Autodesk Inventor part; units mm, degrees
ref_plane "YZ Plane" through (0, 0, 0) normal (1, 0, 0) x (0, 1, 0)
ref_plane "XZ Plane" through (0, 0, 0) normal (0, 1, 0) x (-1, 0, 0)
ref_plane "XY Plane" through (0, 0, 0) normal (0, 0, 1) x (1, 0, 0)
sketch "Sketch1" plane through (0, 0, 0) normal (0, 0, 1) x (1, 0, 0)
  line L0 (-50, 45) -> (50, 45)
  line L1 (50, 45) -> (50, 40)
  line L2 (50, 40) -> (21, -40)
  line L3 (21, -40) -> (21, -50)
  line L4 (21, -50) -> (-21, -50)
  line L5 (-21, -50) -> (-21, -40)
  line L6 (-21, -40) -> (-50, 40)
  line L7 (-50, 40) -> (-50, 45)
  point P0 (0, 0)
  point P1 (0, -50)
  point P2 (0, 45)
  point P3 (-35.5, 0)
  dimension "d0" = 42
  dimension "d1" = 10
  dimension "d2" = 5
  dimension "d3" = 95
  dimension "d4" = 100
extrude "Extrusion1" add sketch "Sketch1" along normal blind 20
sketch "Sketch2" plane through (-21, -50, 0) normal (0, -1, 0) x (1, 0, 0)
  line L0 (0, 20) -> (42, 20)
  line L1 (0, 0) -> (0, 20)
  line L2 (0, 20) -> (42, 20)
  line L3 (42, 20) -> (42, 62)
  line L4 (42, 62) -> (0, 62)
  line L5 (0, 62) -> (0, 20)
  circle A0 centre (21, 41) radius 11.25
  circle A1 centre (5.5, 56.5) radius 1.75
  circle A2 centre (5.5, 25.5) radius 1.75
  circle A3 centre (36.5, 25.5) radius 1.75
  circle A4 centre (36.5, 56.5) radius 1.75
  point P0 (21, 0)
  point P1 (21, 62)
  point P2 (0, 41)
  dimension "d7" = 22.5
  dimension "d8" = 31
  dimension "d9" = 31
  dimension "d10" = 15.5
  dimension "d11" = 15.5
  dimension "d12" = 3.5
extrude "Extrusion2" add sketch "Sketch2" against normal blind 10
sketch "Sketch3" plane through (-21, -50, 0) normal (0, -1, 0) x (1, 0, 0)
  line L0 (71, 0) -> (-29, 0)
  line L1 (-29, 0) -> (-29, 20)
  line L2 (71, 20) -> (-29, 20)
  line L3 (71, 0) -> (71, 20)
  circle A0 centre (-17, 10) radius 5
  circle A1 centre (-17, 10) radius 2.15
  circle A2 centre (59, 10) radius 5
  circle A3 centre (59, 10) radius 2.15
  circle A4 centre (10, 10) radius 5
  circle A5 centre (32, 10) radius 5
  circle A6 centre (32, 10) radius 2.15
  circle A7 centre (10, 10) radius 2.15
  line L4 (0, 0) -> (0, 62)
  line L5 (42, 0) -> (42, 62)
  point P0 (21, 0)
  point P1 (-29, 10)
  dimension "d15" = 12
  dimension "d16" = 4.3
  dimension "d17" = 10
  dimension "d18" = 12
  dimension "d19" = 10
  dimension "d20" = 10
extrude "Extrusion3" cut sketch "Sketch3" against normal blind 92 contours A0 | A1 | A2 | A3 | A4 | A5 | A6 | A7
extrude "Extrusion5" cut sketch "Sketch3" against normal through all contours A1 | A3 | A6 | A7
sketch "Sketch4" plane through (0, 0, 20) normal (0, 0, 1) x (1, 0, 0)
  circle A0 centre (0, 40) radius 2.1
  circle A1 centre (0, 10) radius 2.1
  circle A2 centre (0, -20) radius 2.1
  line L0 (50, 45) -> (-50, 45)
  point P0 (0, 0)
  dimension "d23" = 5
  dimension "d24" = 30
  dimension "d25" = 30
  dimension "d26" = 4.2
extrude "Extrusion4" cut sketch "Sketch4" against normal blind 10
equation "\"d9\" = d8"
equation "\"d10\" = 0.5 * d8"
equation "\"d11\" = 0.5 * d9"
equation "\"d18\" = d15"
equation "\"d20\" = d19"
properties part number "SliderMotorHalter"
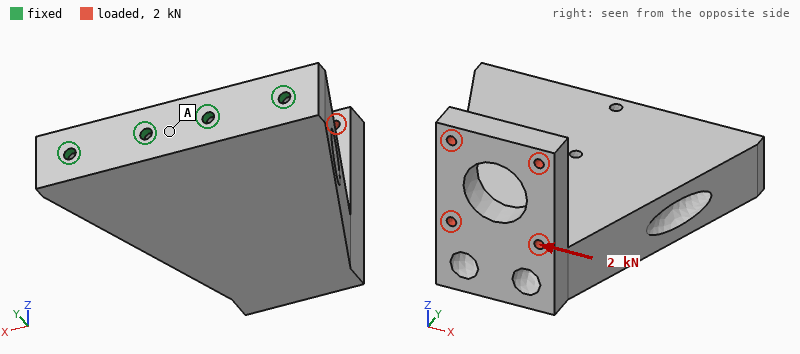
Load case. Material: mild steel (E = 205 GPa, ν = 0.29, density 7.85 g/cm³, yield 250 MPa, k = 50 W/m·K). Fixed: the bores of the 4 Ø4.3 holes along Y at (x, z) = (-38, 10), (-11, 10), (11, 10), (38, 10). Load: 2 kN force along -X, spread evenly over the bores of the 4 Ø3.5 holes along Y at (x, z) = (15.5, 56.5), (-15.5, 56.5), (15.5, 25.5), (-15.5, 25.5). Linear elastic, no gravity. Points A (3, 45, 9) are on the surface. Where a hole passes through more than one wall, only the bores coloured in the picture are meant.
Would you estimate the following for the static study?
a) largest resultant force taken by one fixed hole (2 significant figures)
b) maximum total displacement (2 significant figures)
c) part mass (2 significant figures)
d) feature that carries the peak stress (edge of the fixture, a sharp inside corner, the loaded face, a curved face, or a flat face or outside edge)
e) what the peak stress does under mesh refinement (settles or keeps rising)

2.3 kN
54 µm
980 g
edge of the fixture
keeps rising
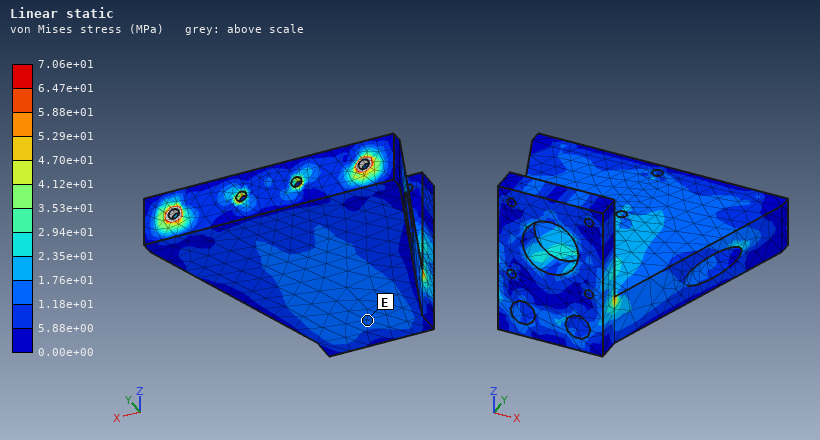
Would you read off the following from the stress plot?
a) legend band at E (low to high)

1.18e+01 to 1.76e+01 MPa
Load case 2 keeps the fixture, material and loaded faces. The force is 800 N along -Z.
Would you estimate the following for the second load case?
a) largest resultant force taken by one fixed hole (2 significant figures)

360 N
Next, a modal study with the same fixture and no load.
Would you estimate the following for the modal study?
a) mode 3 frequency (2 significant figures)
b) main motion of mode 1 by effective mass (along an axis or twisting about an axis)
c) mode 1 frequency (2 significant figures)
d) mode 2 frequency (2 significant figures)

3000 Hz
along Z
510 Hz
2900 Hz
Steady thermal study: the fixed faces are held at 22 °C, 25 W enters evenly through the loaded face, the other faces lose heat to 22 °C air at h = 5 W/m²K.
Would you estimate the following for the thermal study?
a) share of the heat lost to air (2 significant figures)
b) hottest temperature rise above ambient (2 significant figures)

17 %
89 K
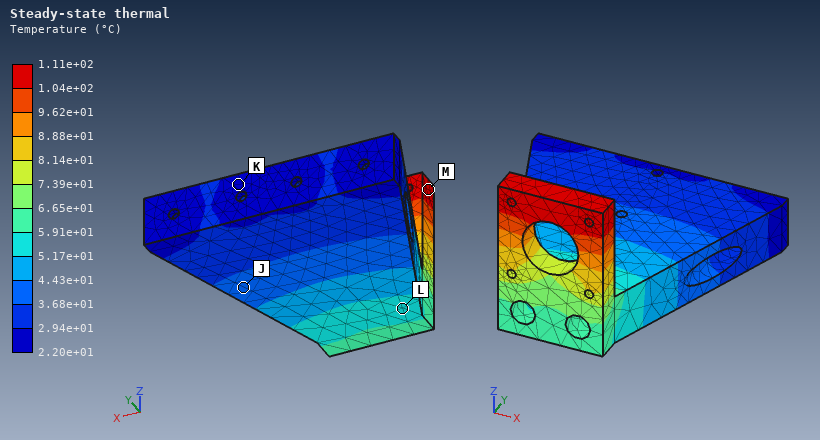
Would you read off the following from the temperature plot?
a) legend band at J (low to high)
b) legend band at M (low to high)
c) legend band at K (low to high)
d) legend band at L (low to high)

3.68e+01 to 4.43e+01 °C
1.04e+02 to 1.11e+02 °C
2.20e+01 to 2.94e+01 °C
5.17e+01 to 5.91e+01 °C
